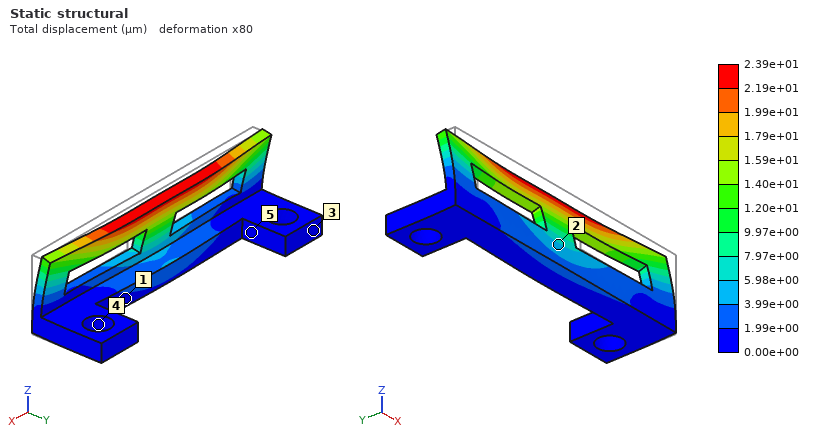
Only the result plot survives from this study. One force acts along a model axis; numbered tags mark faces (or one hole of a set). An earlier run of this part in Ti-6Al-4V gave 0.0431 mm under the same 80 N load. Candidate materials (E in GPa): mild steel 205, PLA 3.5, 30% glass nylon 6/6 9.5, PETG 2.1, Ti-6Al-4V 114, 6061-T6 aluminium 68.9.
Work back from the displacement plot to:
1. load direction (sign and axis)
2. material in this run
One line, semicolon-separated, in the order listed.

+Y; mild steel
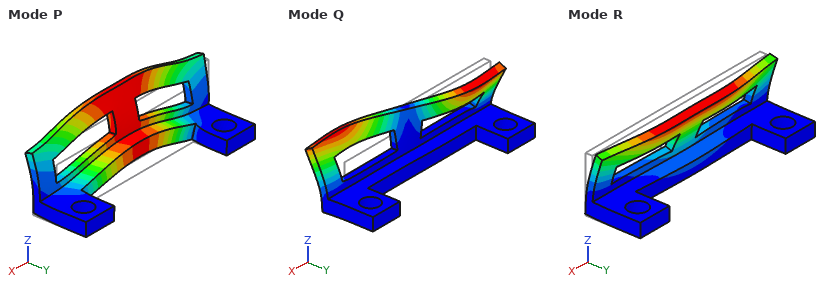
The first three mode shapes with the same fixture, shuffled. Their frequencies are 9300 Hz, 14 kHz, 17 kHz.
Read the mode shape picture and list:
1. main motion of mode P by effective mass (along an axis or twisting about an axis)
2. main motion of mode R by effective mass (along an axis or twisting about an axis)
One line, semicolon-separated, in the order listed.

along Z; along Y
